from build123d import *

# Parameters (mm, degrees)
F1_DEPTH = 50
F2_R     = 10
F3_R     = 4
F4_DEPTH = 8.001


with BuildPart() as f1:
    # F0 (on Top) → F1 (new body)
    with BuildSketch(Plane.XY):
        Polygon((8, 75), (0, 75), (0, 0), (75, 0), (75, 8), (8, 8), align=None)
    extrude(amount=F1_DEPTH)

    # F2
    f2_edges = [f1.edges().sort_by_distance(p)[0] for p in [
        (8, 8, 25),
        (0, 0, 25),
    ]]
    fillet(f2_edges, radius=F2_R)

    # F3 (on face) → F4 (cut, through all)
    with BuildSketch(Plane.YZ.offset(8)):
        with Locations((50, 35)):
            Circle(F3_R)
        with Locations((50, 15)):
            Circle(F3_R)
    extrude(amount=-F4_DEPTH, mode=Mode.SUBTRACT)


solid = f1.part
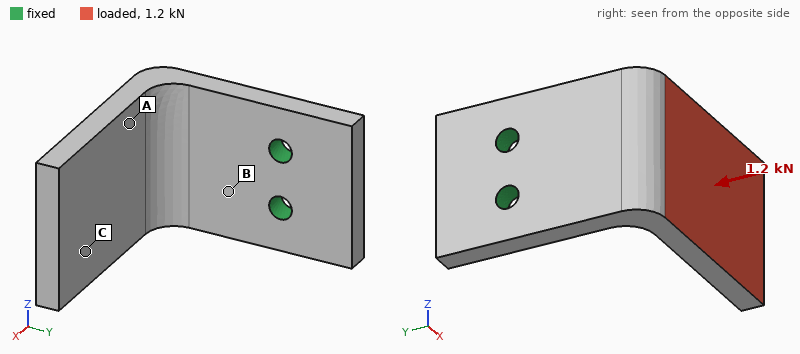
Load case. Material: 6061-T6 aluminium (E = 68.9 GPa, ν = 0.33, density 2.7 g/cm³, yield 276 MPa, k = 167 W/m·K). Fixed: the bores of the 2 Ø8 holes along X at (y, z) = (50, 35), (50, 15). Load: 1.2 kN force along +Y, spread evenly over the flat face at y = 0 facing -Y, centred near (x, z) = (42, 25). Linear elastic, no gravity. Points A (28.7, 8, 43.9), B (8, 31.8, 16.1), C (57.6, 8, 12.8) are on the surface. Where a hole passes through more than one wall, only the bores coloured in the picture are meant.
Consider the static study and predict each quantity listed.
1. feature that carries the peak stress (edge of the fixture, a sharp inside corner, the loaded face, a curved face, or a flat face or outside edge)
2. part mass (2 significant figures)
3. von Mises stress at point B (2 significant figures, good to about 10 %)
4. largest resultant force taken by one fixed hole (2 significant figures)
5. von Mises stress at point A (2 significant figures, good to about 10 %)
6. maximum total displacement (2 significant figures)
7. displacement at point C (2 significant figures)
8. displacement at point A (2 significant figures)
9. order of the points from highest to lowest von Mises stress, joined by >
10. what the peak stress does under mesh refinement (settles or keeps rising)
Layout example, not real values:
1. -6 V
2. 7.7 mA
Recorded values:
1. edge of the fixture
2. 150 g
3. 83 MPa
4. 620 N
5. 35 MPa
6. 1.1 mm
7. 0.81 mm
8. 0.39 mm
9. B > A > C
10. keeps rising
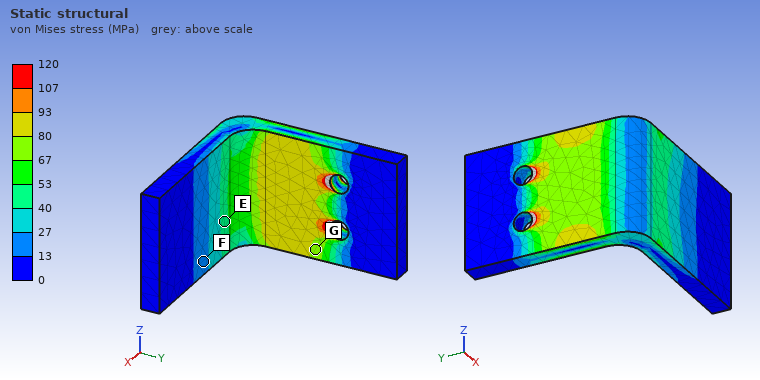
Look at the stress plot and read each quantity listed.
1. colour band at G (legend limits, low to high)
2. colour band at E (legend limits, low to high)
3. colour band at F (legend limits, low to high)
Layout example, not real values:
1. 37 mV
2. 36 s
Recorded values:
1. 67 to 80 MPa
2. 40 to 53 MPa
3. 13 to 27 MPa
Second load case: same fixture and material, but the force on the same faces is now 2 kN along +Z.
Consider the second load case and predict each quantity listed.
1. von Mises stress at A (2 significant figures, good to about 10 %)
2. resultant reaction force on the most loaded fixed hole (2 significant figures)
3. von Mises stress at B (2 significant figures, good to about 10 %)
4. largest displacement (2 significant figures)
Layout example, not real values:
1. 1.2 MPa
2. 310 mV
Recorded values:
1. 20 MPa
2. 4.6 kN
3. 100 MPa
4. 0.74 mm
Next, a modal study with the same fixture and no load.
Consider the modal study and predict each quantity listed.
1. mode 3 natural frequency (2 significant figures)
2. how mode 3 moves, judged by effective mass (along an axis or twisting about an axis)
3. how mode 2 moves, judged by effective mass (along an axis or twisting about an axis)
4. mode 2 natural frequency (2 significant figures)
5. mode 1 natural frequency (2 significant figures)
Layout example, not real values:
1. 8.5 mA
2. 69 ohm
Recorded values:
1. 2200 Hz
2. along X
3. along Z
4. 1100 Hz
5. 690 Hz
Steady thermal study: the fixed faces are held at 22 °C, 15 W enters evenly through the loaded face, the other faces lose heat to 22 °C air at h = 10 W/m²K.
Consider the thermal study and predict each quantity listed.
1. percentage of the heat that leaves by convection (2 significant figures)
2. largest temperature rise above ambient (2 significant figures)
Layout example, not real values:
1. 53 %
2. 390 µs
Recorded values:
1. 6.2 %
2. 16 K
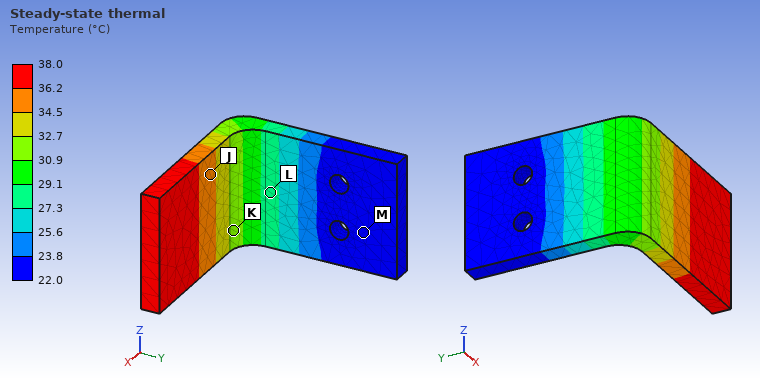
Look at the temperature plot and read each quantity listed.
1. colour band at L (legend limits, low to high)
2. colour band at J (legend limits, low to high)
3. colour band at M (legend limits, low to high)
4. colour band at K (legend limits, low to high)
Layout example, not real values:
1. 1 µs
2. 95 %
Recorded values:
1. 27.3 to 29.1 °C
2. 34.5 to 36.2 °C
3. 22.0 to 23.8 °C
4. 30.9 to 32.7 °C
